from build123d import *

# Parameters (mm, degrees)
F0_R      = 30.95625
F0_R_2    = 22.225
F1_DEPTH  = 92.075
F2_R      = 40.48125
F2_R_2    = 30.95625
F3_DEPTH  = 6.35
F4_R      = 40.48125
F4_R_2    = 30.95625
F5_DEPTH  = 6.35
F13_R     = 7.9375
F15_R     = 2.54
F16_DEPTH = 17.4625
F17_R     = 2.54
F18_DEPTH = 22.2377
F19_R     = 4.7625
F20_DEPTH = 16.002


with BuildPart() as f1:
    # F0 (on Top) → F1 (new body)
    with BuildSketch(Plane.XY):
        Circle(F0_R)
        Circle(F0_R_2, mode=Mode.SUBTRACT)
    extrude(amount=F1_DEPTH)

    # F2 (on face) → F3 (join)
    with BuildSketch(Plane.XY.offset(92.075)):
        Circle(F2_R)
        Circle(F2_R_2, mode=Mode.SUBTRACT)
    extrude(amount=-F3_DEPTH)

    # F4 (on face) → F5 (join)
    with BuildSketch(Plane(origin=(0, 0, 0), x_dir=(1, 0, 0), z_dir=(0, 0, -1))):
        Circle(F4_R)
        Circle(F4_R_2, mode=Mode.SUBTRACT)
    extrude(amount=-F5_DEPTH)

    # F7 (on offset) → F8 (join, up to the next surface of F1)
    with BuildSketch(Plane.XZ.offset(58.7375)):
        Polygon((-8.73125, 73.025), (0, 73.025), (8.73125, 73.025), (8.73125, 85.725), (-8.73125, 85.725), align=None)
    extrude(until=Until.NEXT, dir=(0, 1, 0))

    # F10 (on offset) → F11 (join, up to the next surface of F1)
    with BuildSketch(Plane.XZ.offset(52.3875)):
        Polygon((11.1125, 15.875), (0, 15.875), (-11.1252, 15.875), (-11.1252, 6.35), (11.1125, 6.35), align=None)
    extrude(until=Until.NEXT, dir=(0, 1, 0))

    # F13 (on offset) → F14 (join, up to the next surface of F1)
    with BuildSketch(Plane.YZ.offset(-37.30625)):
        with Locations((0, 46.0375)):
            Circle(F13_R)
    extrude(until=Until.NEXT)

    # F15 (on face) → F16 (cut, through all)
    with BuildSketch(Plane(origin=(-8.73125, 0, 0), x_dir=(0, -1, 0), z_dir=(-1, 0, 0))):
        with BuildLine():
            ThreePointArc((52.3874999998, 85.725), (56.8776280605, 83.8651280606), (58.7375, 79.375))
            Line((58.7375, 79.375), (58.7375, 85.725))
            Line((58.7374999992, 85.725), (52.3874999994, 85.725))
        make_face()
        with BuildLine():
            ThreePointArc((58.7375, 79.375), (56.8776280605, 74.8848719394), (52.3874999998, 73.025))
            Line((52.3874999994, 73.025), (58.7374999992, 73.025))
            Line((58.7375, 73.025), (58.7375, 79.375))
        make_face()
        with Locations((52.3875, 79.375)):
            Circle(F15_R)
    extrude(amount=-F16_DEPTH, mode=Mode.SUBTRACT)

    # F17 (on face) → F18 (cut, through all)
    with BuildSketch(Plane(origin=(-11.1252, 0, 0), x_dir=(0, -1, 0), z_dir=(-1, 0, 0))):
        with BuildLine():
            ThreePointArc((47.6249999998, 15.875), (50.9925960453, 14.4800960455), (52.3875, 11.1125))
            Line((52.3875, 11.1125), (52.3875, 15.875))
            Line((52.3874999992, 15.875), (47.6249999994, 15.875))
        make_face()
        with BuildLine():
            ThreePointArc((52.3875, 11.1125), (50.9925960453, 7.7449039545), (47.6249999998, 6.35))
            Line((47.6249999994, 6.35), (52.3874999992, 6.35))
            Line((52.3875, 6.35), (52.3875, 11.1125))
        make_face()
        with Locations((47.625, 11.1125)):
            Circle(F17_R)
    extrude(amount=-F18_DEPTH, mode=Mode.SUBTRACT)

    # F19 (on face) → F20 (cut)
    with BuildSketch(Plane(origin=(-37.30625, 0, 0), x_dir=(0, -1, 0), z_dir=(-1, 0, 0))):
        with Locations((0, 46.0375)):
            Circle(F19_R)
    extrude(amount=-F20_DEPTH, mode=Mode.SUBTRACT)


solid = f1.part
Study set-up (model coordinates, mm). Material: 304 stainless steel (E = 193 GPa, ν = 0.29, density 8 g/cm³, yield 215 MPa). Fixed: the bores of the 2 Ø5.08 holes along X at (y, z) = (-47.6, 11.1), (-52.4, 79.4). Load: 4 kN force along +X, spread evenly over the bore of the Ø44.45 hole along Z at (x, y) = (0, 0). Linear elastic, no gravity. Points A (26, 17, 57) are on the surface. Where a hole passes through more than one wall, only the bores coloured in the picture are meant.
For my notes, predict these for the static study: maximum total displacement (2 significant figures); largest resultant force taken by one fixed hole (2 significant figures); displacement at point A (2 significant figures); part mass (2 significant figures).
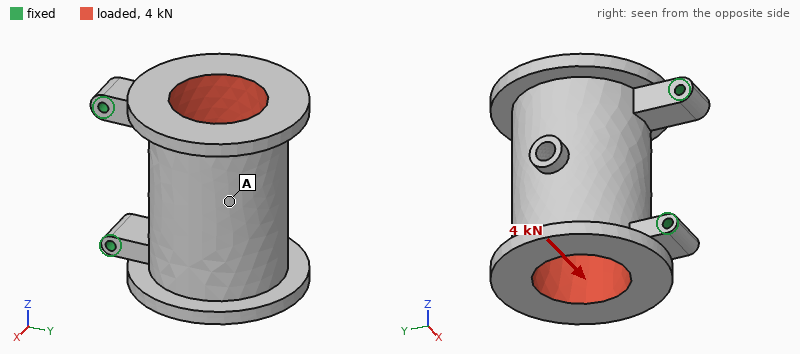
0.11 mm
2.0 kN
0.088 mm
1.4 kg
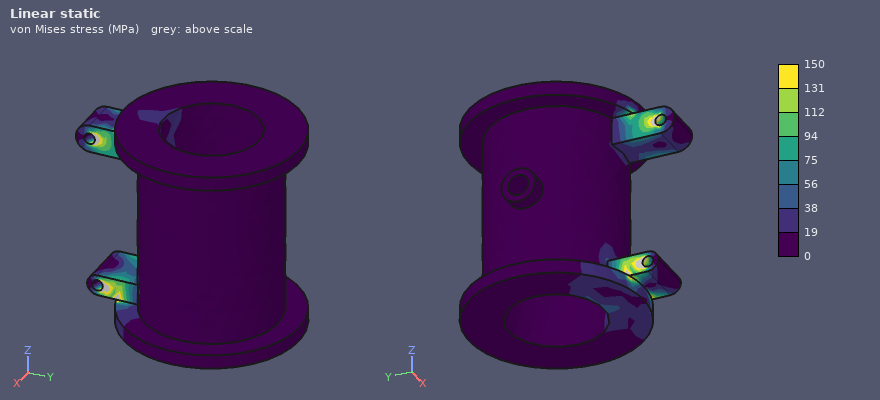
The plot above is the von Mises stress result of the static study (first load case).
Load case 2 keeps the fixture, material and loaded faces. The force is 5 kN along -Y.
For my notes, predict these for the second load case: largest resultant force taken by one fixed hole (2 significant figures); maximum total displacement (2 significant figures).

2.6 kN
5.9 µm
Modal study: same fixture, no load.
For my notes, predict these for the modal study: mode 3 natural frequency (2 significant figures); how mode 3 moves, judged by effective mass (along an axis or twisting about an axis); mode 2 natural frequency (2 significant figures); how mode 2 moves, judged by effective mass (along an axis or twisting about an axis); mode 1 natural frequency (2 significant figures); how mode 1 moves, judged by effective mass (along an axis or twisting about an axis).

3800 Hz
twisting about Y
2400 Hz
along Z
970 Hz
along X
